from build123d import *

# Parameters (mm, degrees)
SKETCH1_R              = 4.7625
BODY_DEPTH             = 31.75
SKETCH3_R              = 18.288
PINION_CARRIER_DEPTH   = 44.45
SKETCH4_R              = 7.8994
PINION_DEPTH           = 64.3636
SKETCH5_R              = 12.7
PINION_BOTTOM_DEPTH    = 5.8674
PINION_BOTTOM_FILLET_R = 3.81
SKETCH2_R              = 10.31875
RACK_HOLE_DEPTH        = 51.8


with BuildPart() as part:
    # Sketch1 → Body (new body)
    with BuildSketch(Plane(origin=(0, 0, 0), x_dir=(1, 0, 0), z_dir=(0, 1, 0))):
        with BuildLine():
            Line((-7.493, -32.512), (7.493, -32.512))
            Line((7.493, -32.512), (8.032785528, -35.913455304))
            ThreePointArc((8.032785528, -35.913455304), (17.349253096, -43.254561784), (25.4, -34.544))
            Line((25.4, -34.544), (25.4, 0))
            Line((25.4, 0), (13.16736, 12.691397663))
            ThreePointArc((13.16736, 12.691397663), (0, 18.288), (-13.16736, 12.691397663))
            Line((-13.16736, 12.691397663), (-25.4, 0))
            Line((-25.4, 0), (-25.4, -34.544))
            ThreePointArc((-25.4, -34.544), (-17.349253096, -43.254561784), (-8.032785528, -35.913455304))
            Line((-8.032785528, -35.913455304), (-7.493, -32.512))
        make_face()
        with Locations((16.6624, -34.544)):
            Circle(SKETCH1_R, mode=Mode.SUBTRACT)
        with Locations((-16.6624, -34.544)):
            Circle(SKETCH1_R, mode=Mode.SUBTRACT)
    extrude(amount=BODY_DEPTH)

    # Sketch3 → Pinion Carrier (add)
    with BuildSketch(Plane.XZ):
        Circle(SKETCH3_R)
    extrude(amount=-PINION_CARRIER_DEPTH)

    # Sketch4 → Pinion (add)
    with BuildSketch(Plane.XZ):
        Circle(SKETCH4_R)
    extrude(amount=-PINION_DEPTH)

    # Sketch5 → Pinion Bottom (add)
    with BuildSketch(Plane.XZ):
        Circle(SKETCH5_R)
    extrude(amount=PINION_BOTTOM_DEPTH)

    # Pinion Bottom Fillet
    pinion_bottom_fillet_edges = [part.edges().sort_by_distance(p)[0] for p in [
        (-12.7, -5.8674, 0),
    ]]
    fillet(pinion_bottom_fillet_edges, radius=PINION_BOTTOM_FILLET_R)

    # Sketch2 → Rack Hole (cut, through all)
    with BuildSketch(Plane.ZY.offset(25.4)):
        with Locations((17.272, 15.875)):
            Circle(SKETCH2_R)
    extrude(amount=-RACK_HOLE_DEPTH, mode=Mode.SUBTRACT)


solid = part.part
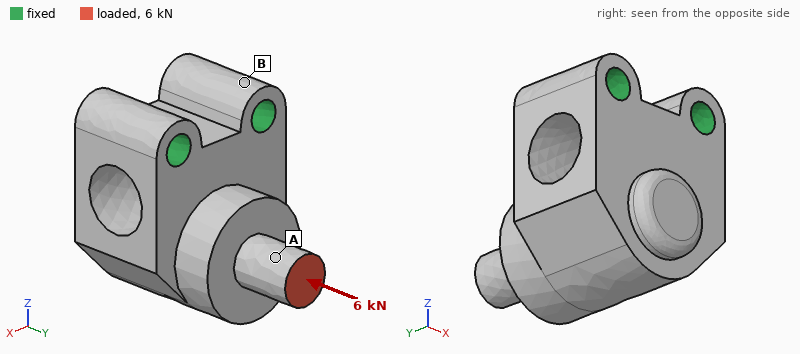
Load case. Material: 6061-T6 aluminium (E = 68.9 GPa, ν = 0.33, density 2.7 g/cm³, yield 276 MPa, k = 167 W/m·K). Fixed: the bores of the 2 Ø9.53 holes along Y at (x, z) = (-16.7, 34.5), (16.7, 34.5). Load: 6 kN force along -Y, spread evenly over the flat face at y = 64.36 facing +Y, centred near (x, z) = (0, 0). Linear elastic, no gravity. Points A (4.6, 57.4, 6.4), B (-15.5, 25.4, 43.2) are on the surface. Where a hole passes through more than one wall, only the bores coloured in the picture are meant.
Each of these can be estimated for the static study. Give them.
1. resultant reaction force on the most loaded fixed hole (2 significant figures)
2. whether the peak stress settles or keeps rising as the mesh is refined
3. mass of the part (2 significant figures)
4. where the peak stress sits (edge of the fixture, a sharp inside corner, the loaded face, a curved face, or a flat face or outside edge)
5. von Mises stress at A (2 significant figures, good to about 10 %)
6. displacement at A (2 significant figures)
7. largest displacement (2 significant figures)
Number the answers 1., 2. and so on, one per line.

1. 3.0 kN
2. keeps rising
3. 210 g
4. edge of the fixture
5. 30 MPa
6. 52 µm
7. 68 µm
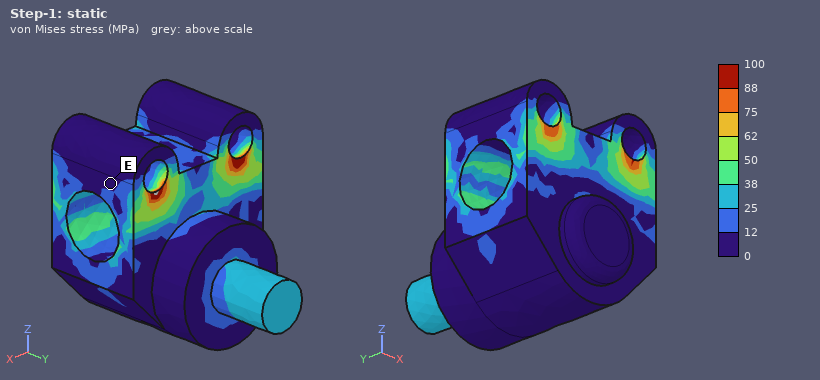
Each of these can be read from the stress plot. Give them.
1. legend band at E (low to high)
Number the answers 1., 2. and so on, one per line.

1. 0 to 12 MPa
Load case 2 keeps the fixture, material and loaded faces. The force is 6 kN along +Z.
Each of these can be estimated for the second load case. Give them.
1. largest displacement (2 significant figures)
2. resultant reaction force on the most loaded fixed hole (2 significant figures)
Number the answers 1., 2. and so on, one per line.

1. 0.25 mm
2. 3.4 kN
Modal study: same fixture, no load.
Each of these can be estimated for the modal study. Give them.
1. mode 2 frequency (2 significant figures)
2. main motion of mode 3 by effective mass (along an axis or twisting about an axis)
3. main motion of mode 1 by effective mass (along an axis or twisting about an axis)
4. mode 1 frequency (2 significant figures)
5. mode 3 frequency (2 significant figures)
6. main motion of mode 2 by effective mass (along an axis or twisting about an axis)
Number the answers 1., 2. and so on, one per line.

1. 6800 Hz
2. along X
3. along Y
4. 4700 Hz
5. 8900 Hz
6. along X
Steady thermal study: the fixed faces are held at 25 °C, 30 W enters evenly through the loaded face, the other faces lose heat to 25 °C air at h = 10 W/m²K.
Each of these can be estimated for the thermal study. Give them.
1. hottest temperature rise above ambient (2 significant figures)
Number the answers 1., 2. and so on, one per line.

1. 30 K
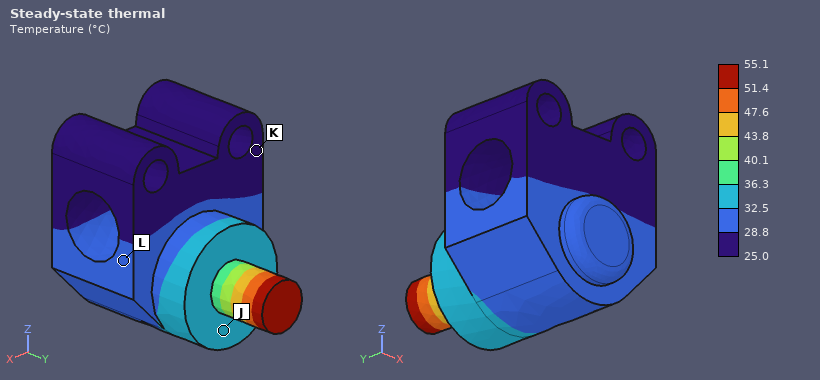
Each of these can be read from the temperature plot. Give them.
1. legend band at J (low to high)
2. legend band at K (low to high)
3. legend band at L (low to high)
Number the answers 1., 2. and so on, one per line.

1. 32.5 to 36.3 °C
2. 25.0 to 28.8 °C
3. 28.8 to 32.5 °C
